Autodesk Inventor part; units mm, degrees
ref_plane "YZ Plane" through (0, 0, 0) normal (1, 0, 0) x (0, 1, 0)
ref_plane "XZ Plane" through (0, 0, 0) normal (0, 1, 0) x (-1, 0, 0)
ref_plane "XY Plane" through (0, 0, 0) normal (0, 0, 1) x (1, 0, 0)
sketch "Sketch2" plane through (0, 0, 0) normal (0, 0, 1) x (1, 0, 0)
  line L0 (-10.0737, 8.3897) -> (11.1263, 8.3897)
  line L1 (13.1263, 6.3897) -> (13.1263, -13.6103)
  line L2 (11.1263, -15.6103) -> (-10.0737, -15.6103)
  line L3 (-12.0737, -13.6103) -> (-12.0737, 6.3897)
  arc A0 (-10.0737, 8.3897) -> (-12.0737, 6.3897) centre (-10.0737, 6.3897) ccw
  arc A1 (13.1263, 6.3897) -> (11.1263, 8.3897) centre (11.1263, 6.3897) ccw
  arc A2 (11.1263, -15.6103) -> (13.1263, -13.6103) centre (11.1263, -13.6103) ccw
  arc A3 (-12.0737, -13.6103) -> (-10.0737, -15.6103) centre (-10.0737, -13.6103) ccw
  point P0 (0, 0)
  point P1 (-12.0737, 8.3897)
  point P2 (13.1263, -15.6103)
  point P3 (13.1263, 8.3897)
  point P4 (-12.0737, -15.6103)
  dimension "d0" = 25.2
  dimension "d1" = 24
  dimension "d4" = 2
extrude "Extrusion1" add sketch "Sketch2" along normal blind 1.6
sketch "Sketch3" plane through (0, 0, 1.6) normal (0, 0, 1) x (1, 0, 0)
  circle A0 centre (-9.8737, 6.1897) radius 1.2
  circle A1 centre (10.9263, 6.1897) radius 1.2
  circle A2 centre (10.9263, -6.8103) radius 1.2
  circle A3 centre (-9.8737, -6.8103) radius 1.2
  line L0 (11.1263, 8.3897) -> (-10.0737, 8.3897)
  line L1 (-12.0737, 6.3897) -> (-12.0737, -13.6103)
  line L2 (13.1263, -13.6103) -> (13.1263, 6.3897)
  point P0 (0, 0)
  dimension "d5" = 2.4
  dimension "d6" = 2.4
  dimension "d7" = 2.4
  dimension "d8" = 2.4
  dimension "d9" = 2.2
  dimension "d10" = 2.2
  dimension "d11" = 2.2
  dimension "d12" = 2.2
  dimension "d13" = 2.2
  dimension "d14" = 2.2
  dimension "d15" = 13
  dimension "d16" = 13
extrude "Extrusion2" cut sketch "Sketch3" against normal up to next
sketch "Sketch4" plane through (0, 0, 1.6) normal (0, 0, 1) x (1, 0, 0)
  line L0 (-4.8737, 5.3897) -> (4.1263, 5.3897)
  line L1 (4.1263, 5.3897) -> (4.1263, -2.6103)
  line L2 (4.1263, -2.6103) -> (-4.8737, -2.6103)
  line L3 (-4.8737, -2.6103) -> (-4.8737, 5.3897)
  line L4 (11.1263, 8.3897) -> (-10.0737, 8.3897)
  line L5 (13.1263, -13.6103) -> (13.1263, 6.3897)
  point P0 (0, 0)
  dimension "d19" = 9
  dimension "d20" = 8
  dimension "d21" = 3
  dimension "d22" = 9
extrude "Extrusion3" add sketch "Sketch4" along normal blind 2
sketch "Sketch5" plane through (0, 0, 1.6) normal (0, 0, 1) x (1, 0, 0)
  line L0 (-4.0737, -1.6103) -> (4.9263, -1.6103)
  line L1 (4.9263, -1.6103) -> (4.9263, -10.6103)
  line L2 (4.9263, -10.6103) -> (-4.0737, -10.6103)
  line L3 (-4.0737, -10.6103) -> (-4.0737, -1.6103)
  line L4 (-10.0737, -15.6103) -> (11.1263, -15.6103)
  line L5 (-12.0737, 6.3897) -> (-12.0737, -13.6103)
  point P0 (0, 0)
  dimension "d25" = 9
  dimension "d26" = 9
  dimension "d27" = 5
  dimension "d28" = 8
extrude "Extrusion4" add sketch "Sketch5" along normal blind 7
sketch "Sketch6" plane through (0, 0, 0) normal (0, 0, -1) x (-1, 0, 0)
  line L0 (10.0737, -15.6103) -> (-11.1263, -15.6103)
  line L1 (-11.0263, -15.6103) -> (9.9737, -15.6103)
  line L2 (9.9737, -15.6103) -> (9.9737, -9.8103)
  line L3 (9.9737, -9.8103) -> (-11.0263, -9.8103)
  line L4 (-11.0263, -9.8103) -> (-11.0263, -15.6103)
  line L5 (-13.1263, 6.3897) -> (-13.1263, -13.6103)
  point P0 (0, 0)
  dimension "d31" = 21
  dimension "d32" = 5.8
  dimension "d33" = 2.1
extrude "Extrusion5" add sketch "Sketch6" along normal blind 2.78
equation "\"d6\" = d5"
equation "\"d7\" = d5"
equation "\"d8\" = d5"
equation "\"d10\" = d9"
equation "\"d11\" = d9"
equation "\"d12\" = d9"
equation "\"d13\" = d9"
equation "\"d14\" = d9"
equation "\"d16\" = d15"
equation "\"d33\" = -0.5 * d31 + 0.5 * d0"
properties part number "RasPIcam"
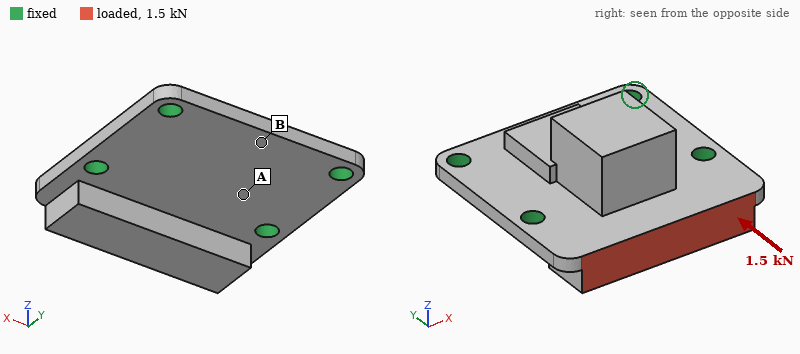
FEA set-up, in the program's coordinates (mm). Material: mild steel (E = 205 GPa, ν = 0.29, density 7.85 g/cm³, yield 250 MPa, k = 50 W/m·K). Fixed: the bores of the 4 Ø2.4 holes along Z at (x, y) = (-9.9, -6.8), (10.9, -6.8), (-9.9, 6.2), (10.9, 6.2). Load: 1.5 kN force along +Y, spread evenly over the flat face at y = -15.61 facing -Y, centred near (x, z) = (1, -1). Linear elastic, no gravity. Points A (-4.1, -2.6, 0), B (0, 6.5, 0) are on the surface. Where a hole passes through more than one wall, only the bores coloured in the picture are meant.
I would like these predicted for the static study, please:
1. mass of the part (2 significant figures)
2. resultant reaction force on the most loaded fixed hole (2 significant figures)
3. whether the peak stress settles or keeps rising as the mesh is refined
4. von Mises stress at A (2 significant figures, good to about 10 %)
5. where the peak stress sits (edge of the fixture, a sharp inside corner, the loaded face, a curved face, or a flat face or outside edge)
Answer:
15 g
610 N
keeps rising
47 MPa
edge of the fixture
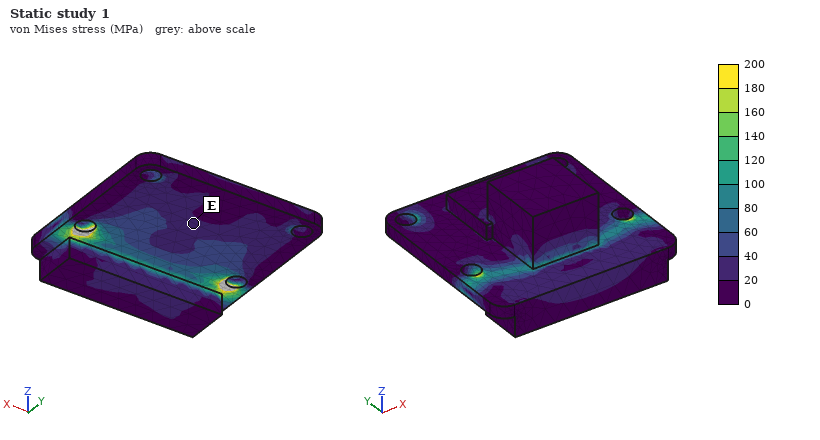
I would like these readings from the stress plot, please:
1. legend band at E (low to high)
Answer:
20 to 40 MPa
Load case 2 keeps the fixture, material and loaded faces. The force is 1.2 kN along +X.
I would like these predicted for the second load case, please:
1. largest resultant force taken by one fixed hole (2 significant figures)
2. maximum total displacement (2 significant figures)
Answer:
730 N
4.3 µm
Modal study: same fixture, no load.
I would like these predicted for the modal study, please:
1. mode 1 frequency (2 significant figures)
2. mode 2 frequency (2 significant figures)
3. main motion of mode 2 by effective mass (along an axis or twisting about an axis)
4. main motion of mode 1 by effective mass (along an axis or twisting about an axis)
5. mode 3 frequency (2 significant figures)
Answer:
12 kHz
18 kHz
along Z
along Z
26 kHz
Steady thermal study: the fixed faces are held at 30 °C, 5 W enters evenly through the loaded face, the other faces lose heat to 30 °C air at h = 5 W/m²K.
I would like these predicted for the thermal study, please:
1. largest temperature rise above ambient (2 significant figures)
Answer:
19 K
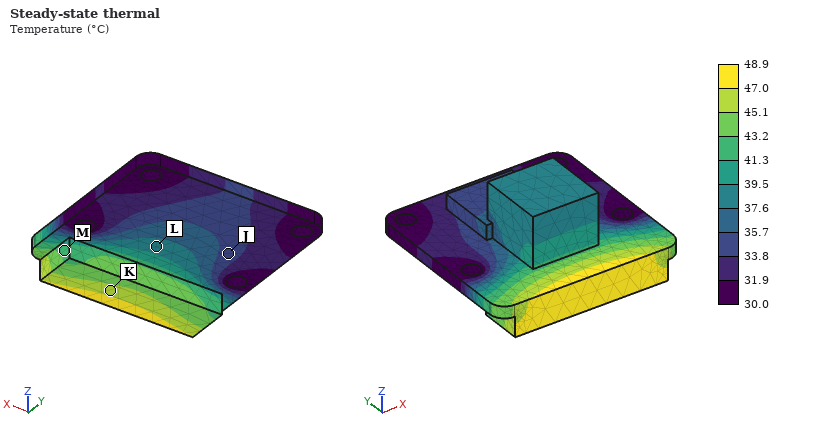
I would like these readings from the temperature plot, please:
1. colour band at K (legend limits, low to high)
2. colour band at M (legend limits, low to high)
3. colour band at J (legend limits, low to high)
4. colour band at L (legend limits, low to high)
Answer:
45.1 to 47.0 °C
41.3 to 43.2 °C
33.8 to 35.7 °C
37.6 to 39.5 °C
